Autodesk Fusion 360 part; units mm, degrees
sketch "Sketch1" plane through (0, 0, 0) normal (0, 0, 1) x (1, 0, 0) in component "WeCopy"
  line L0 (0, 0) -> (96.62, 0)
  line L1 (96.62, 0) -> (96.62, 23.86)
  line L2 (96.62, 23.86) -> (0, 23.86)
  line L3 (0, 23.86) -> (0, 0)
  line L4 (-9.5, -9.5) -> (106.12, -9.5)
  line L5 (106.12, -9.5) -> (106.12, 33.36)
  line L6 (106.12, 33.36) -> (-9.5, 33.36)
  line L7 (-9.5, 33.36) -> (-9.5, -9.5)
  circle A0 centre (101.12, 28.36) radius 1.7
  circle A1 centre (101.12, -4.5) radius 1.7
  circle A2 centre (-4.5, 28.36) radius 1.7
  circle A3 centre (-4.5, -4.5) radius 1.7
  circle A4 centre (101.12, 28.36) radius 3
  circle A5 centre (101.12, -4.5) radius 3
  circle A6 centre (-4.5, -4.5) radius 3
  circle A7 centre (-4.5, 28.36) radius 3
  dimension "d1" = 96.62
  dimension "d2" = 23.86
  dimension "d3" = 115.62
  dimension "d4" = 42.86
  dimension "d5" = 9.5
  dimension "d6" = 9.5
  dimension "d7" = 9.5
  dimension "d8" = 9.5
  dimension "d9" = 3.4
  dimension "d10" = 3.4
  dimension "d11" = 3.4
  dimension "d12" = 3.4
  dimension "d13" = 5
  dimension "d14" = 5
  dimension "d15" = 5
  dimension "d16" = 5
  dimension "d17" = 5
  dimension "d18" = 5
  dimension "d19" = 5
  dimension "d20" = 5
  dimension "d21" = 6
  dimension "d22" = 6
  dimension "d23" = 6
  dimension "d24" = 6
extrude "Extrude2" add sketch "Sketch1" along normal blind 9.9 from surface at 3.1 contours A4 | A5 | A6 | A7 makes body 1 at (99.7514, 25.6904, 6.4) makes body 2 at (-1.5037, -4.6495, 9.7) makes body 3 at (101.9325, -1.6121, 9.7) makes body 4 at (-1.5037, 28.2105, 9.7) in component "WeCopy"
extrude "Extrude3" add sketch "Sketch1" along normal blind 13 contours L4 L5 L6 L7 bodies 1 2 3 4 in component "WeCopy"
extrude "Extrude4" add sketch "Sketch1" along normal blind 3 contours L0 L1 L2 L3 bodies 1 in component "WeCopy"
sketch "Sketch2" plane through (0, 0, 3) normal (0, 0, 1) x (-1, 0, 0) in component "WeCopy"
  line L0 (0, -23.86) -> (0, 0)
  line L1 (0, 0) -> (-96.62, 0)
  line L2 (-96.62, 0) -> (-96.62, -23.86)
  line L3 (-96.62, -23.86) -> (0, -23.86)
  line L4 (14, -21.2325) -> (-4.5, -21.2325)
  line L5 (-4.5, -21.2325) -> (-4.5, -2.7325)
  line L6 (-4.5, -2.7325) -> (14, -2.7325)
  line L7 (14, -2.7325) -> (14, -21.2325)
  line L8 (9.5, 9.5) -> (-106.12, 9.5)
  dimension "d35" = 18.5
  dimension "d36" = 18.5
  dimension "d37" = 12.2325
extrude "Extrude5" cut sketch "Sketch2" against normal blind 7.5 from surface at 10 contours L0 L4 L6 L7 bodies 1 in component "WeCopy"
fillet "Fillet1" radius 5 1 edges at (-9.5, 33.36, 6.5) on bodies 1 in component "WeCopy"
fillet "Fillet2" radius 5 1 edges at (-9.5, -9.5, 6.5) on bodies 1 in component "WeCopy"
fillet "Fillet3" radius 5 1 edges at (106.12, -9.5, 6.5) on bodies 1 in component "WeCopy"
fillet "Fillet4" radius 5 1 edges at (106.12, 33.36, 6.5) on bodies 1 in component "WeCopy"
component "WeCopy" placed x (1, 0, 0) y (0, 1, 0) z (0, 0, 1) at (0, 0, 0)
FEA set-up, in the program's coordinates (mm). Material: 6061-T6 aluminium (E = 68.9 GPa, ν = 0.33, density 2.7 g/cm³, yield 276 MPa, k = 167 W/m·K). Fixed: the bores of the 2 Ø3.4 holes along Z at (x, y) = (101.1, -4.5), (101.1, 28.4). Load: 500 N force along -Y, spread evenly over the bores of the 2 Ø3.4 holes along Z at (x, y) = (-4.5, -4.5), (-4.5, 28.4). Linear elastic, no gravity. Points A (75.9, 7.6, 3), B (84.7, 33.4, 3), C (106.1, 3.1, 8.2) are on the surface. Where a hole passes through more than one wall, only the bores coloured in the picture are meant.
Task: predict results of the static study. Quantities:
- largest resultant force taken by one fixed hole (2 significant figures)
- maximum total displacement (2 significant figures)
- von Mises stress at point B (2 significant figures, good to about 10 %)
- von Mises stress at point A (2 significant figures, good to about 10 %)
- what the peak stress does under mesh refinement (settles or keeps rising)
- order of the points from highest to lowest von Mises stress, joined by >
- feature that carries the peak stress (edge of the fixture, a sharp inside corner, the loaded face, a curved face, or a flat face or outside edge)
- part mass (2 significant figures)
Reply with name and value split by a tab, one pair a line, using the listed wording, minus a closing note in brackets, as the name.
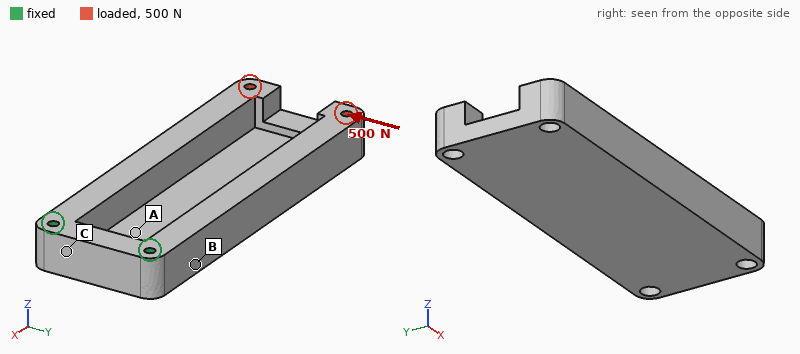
largest resultant force taken by one fixed hole	1.5 kN
maximum total displacement	0.14 mm
von Mises stress at point B	19 MPa
von Mises stress at point A	12 MPa
what the peak stress does under mesh refinement	keeps rising
order of the points from highest to lowest von Mises stress, joined by >	B > A > C
feature that carries the peak stress	edge of the fixture
part mass	110 g
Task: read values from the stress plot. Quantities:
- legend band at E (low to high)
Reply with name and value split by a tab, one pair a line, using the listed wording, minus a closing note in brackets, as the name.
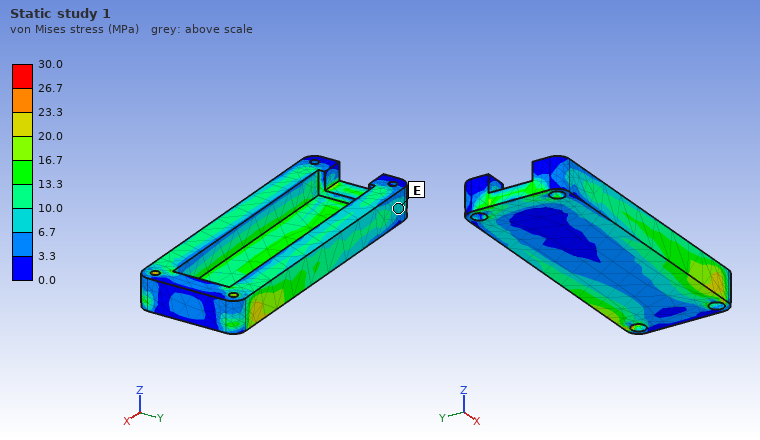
legend band at E	6.7 to 10.0 MPa
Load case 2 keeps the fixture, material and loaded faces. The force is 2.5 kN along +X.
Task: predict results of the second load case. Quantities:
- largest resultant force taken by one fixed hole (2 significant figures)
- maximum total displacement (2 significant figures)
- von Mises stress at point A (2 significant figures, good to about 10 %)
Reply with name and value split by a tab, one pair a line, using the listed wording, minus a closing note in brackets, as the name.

largest resultant force taken by one fixed hole	1.3 kN
maximum total displacement	0.11 mm
von Mises stress at point A	4.3 MPa
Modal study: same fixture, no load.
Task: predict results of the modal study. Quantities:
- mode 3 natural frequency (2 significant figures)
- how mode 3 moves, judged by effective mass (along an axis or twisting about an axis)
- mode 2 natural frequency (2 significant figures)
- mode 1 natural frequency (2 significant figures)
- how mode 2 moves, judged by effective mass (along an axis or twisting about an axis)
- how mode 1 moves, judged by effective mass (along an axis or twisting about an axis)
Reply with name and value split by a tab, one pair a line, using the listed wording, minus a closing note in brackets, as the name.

mode 3 natural frequency	3100 Hz
how mode 3 moves, judged by effective mass	along Y
mode 2 natural frequency	1700 Hz
mode 1 natural frequency	780 Hz
how mode 2 moves, judged by effective mass	along Y
how mode 1 moves, judged by effective mass	along Z
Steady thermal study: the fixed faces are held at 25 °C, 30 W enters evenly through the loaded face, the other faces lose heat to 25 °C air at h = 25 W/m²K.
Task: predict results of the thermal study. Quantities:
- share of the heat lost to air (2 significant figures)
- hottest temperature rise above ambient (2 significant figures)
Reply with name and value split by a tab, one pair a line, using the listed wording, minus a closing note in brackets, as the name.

share of the heat lost to air	30 %
hottest temperature rise above ambient	50 K
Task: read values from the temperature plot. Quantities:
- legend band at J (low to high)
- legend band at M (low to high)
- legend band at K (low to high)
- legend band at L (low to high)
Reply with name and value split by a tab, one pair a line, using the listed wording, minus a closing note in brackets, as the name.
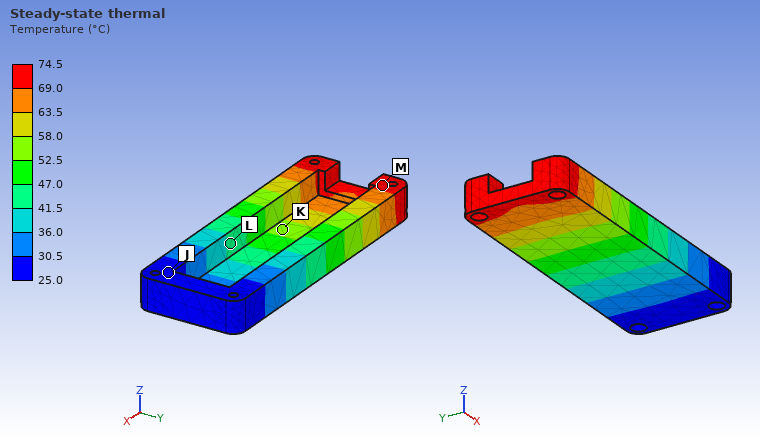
legend band at J	25.0 to 30.5 °C
legend band at M	69.0 to 74.5 °C
legend band at K	52.5 to 58.0 °C
legend band at L	41.5 to 47.0 °C
